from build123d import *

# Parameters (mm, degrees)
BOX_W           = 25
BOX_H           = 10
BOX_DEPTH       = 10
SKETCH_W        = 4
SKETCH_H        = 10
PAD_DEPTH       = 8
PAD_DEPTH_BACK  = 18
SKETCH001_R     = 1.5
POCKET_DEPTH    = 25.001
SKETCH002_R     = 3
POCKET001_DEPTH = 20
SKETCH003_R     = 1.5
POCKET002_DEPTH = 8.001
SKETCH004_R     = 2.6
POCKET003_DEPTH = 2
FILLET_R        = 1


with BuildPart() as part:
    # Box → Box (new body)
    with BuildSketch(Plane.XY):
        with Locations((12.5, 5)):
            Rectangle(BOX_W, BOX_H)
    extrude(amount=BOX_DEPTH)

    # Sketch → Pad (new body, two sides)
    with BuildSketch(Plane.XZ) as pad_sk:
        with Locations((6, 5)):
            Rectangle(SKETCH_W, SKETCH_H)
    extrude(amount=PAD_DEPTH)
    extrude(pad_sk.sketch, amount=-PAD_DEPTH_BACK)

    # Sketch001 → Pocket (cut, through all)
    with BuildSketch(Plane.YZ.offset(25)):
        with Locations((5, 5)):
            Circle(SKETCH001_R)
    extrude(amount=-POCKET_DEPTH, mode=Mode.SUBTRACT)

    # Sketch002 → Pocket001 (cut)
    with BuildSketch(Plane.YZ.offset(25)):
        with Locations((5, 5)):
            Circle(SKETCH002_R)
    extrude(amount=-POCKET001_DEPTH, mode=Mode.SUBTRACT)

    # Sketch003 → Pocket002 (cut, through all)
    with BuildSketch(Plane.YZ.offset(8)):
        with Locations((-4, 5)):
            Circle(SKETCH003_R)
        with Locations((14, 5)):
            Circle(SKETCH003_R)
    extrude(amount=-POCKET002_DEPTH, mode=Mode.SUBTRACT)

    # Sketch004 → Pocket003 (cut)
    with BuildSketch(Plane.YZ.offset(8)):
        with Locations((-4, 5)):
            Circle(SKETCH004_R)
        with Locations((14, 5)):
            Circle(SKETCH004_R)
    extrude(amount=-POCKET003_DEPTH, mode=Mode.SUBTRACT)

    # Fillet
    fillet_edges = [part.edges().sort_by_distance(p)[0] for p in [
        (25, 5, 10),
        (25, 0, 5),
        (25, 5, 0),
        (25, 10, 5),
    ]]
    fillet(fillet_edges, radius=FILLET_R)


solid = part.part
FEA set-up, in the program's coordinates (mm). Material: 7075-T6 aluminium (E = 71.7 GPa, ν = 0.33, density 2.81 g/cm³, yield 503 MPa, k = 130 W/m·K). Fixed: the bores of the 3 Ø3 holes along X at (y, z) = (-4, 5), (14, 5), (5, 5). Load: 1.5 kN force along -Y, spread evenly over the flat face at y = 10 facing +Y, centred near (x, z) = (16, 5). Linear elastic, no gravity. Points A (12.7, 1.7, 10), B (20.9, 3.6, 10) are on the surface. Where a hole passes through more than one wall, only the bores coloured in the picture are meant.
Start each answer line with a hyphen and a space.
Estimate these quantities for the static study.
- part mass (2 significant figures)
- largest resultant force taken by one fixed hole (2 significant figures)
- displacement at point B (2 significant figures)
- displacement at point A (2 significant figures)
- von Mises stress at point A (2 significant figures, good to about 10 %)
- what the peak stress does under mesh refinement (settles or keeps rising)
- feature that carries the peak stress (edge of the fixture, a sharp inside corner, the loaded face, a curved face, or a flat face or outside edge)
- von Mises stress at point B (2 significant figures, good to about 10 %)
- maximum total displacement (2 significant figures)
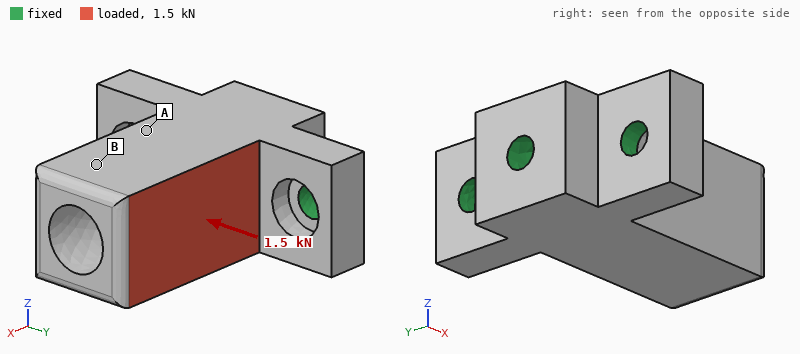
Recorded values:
- 6.8 g
- 1.2 kN
- 40 µm
- 17 µm
- 41 MPa
- keeps rising
- edge of the fixture
- 16 MPa
- 53 µm
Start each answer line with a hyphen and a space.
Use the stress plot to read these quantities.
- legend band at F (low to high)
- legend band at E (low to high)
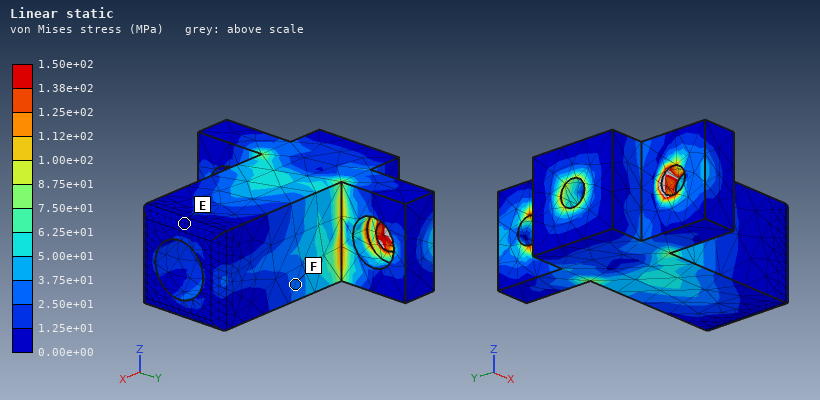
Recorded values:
- 2.50e+01 to 3.75e+01 MPa
- 0.00e+00 to 1.25e+01 MPa
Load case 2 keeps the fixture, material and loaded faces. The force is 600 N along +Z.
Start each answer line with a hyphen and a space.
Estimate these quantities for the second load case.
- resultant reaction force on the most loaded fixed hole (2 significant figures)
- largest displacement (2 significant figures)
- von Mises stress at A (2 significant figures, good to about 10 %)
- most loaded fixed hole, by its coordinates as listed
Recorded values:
- 400 N
- 47 µm
- 20 MPa
- (14, 5)
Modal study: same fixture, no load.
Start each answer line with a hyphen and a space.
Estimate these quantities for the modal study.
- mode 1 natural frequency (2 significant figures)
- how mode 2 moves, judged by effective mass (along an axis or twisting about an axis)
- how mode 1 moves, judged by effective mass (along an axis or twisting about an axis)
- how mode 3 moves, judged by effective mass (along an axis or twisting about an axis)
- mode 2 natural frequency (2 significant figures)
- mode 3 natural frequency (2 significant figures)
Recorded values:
- 12 kHz
- along Y
- along Z
- twisting about X
- 17 kHz
- 36 kHz
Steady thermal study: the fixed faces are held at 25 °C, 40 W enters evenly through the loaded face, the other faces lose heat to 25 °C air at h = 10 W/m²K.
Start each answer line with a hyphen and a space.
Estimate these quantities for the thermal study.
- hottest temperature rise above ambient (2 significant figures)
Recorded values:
- 60 K
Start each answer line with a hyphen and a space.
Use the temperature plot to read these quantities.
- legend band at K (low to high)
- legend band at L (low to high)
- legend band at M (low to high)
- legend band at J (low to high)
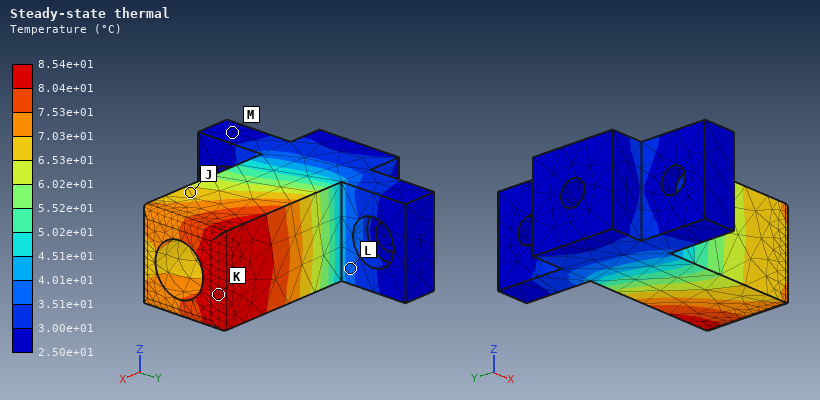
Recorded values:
- 8.04e+01 to 8.54e+01 °C
- 3.51e+01 to 4.01e+01 °C
- 2.50e+01 to 3.00e+01 °C
- 6.53e+01 to 7.03e+01 °C
